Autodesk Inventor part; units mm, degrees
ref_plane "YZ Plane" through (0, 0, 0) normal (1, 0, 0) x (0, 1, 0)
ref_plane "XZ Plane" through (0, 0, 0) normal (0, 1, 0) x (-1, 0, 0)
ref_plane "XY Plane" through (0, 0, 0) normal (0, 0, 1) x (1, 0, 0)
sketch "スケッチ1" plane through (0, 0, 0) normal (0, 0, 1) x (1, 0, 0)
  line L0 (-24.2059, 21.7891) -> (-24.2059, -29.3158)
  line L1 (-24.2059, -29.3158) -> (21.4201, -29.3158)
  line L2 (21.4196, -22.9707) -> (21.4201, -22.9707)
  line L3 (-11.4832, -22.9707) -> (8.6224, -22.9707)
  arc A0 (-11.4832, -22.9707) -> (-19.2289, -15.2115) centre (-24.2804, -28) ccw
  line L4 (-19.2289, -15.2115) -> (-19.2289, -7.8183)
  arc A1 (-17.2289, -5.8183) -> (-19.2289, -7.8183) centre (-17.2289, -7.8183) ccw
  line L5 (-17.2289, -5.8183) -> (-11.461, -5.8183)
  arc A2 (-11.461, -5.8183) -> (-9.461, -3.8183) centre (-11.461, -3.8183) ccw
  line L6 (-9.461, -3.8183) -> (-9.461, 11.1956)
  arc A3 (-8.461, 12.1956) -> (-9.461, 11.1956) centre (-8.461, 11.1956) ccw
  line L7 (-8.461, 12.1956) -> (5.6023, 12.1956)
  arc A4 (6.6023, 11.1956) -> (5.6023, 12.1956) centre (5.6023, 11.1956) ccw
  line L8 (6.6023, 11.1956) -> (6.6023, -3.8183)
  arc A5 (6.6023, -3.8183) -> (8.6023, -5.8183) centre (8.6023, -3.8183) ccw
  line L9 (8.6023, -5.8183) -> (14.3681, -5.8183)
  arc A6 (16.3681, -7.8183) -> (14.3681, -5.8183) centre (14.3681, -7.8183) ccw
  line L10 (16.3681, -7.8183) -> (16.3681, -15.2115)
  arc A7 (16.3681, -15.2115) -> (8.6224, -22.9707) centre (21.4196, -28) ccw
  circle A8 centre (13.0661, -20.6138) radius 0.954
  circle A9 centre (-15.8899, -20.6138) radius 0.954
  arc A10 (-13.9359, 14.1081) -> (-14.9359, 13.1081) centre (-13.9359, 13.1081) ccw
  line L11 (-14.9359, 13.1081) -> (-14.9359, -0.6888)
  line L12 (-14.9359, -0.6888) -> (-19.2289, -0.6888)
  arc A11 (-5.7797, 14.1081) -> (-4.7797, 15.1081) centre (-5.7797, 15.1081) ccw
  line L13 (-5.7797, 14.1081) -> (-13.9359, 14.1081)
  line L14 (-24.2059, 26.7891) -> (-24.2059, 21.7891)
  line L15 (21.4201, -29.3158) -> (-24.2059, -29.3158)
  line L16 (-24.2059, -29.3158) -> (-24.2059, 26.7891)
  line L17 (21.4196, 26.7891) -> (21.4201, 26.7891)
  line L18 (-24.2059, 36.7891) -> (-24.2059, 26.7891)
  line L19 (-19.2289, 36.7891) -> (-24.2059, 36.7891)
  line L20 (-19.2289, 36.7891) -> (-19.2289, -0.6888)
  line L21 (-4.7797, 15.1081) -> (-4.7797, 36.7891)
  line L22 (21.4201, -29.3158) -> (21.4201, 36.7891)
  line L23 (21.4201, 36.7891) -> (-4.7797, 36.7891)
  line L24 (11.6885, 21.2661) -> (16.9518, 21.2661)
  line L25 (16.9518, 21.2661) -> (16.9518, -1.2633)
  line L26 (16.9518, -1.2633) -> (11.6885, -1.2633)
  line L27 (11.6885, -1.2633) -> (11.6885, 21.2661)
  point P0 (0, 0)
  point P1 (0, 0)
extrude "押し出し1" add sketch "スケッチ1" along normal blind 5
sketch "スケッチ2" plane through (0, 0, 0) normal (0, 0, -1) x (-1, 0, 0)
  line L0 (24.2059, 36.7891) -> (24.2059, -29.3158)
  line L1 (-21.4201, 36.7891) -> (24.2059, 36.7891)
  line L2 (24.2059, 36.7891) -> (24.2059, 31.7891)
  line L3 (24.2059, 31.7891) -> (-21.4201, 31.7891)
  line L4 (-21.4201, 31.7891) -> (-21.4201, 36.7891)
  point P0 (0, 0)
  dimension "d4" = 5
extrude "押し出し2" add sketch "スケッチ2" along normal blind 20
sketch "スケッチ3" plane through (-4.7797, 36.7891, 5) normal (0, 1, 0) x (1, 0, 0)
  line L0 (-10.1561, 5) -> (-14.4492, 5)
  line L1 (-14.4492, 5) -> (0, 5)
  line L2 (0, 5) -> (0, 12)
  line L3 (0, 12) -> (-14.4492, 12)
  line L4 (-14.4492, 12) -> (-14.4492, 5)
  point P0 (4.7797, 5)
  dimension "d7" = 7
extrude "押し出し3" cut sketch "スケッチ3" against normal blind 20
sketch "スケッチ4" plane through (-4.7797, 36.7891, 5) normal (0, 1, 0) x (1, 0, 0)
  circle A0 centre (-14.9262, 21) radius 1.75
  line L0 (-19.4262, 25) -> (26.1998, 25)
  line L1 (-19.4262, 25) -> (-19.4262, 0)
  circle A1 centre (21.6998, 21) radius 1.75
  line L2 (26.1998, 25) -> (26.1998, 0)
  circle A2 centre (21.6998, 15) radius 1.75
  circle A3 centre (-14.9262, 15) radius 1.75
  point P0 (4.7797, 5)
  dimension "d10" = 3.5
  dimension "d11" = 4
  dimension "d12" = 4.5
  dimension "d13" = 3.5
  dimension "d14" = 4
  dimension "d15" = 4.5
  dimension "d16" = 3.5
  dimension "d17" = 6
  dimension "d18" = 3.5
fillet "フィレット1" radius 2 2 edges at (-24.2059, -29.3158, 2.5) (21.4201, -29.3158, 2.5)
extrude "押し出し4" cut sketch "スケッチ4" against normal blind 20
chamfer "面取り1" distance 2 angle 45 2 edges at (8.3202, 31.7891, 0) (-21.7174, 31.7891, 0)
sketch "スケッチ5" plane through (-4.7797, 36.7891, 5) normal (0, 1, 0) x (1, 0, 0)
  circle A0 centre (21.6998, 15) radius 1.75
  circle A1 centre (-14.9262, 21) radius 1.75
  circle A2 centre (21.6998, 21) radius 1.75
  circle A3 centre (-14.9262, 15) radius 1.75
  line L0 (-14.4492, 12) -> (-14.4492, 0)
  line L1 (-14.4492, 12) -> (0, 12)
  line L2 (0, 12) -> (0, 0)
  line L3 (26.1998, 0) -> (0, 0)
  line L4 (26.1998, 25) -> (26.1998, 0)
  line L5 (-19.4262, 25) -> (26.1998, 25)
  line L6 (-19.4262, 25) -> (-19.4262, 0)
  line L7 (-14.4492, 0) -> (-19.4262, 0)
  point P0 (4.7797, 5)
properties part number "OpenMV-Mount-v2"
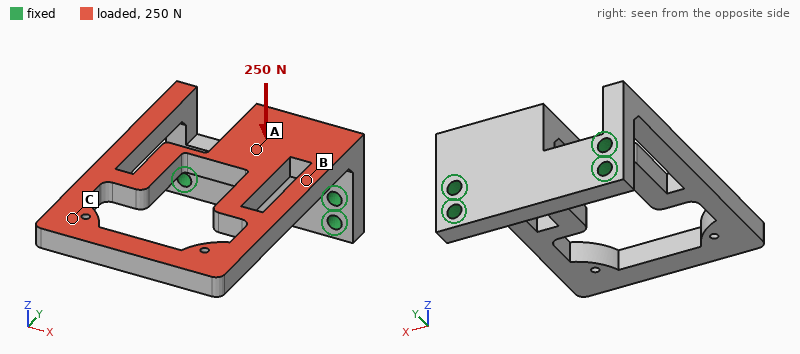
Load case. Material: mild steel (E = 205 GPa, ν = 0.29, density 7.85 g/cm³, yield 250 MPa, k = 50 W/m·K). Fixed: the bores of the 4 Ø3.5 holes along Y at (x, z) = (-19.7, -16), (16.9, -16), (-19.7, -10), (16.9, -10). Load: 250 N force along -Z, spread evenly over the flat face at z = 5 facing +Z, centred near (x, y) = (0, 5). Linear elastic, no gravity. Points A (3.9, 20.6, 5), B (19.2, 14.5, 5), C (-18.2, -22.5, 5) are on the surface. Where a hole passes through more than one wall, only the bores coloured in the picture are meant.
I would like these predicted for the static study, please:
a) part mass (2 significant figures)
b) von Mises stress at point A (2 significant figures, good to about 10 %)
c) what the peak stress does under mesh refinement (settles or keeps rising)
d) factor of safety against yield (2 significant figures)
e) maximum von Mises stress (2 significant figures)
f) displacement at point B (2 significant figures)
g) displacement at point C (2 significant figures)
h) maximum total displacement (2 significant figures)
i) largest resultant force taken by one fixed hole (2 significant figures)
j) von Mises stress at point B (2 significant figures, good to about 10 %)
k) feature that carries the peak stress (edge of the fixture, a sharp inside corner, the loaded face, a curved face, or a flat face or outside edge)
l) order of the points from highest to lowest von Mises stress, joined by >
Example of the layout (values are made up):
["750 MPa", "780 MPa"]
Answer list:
["97 g", "30 MPa", "settles", "1.4", "180 MPa", "0.039 mm", "0.22 mm", "0.26 mm", "250 N", "48 MPa", "a curved face", "B > A > C"]
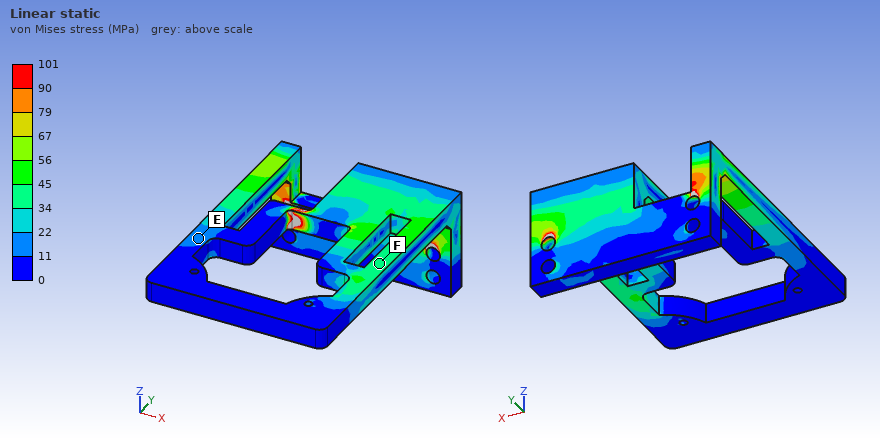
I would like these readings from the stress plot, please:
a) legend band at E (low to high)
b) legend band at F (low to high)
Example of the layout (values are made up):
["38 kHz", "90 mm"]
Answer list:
["11 to 22 MPa", "34 to 45 MPa"]
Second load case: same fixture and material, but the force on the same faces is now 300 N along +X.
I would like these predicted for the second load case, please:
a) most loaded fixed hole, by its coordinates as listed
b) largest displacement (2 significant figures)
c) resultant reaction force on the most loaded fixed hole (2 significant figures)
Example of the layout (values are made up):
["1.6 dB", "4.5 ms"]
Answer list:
["(16.9, -10)", "27 µm", "370 N"]
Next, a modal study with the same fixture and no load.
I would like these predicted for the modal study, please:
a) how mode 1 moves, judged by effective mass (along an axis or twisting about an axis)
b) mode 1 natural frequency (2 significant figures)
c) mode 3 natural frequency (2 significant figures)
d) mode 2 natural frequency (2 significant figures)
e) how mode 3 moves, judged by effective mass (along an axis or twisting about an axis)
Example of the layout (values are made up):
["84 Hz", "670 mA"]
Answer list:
["along Z", "750 Hz", "2500 Hz", "1800 Hz", "along X"]
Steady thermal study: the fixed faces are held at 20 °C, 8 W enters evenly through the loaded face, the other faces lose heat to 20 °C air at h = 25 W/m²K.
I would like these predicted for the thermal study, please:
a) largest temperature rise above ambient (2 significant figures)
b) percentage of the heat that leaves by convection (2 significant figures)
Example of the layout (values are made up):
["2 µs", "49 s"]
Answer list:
["38 K", "33 %"]
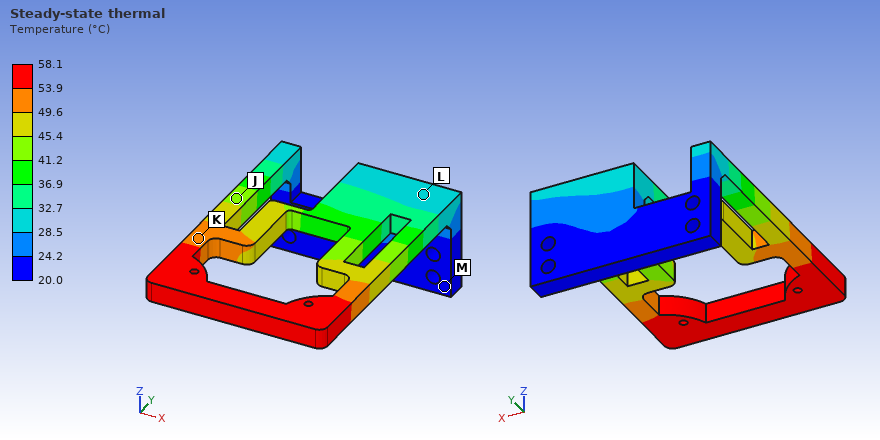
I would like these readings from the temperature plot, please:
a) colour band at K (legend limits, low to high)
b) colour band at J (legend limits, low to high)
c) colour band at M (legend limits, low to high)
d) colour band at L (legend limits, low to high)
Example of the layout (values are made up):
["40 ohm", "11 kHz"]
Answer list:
["49.6 to 53.9 °C", "41.2 to 45.4 °C", "20.0 to 24.2 °C", "28.5 to 32.7 °C"]
